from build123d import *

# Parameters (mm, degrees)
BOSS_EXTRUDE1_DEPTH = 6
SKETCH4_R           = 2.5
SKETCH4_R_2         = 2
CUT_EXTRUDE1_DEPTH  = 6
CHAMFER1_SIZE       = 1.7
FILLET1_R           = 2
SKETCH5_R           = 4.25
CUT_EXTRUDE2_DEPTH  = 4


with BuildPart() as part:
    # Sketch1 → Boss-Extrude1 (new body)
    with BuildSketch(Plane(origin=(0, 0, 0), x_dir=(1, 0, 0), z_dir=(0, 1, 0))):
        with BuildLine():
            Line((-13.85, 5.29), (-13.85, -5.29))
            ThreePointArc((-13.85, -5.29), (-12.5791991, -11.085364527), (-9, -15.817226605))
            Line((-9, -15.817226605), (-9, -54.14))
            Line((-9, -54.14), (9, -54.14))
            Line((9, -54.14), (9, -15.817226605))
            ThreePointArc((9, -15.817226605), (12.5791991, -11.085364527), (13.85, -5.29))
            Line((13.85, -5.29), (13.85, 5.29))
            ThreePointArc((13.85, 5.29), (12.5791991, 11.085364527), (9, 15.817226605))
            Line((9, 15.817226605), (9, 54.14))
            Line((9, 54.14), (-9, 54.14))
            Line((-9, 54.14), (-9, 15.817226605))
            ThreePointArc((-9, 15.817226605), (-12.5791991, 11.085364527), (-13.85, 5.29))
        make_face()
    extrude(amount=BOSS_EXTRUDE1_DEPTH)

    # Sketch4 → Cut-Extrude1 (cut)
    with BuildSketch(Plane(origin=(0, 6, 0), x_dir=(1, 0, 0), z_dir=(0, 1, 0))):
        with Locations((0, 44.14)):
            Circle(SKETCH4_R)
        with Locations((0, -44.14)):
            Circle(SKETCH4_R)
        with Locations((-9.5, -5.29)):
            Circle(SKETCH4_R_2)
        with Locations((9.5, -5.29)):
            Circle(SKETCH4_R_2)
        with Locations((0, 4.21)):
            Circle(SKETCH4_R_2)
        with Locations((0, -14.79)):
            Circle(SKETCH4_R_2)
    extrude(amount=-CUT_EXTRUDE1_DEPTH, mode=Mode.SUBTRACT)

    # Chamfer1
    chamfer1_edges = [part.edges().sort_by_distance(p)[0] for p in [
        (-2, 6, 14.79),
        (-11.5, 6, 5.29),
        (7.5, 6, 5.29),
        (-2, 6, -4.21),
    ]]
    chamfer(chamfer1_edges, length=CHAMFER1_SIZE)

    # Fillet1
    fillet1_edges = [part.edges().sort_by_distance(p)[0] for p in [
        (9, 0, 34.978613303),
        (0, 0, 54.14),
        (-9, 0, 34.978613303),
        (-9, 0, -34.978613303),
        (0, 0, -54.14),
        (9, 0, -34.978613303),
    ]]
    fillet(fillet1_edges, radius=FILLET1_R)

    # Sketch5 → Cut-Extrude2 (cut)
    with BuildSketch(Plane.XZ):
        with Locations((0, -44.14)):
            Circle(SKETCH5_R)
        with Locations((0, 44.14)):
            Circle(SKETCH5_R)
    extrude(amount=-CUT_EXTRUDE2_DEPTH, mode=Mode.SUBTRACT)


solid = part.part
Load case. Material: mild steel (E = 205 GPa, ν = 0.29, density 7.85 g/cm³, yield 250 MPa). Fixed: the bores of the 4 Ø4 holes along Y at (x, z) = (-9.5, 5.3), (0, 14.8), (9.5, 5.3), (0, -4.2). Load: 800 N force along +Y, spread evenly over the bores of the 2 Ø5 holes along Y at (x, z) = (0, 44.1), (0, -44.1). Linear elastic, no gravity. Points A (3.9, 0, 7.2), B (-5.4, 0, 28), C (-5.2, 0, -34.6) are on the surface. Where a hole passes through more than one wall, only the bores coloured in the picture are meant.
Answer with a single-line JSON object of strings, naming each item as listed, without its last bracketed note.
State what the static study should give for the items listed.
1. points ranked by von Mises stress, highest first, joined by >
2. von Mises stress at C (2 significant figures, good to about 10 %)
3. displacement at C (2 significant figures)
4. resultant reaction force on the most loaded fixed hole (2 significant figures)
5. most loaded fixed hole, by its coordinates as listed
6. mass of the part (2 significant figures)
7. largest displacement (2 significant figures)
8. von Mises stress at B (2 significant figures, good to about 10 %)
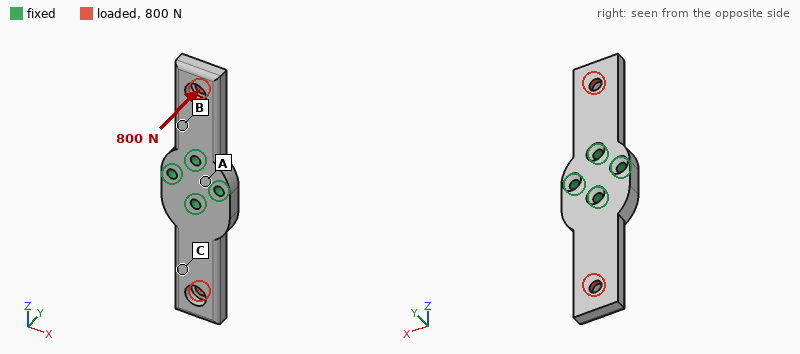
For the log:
{"points ranked by von Mises stress, highest first, joined by >": "B > C > A", "von Mises stress at C": "39 MPa", "displacement at C": "0.082 mm", "resultant reaction force on the most loaded fixed hole": "1.2 kN", "most loaded fixed hole, by its coordinates as listed": "(0, -4.2)", "mass of the part": "95 g", "largest displacement": "0.17 mm", "von Mises stress at B": "62 MPa"}
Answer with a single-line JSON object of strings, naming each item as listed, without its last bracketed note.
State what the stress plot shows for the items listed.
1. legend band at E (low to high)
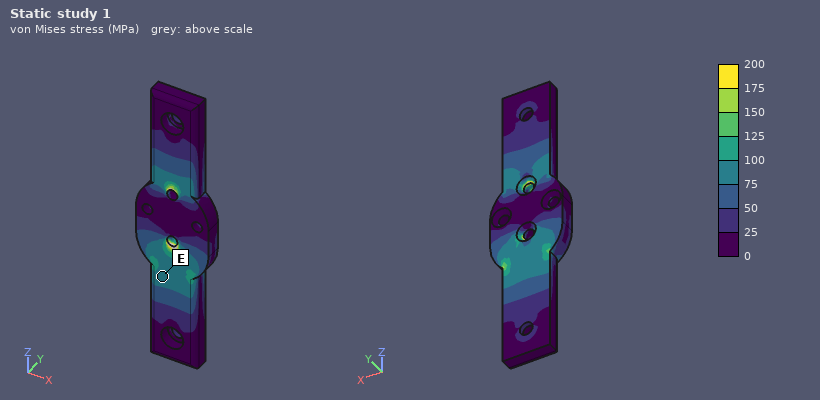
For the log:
{"legend band at E": "75 to 100 MPa"}
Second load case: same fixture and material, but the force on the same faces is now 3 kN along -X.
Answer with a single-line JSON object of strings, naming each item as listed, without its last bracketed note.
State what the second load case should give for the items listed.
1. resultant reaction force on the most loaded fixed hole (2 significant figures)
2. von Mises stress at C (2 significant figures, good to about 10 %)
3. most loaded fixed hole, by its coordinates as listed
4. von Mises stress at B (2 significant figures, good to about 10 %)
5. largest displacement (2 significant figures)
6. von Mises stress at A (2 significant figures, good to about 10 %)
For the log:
{"resultant reaction force on the most loaded fixed hole": "1.8 kN", "von Mises stress at C": "20 MPa", "most loaded fixed hole, by its coordinates as listed": "(0, -4.2)", "von Mises stress at B": "46 MPa", "largest displacement": "79 µm", "von Mises stress at A": "28 MPa"}
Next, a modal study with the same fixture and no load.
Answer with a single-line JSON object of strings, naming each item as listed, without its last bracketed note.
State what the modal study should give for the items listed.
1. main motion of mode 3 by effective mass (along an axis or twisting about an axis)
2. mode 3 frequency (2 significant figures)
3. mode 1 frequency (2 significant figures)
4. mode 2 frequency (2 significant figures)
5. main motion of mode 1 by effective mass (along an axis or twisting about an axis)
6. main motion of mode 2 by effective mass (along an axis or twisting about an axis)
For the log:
{"main motion of mode 3 by effective mass": "along X", "mode 3 frequency": "6200 Hz", "mode 1 frequency": "2100 Hz", "mode 2 frequency": "3200 Hz", "main motion of mode 1 by effective mass": "along Y", "main motion of mode 2 by effective mass": "along Y"}
